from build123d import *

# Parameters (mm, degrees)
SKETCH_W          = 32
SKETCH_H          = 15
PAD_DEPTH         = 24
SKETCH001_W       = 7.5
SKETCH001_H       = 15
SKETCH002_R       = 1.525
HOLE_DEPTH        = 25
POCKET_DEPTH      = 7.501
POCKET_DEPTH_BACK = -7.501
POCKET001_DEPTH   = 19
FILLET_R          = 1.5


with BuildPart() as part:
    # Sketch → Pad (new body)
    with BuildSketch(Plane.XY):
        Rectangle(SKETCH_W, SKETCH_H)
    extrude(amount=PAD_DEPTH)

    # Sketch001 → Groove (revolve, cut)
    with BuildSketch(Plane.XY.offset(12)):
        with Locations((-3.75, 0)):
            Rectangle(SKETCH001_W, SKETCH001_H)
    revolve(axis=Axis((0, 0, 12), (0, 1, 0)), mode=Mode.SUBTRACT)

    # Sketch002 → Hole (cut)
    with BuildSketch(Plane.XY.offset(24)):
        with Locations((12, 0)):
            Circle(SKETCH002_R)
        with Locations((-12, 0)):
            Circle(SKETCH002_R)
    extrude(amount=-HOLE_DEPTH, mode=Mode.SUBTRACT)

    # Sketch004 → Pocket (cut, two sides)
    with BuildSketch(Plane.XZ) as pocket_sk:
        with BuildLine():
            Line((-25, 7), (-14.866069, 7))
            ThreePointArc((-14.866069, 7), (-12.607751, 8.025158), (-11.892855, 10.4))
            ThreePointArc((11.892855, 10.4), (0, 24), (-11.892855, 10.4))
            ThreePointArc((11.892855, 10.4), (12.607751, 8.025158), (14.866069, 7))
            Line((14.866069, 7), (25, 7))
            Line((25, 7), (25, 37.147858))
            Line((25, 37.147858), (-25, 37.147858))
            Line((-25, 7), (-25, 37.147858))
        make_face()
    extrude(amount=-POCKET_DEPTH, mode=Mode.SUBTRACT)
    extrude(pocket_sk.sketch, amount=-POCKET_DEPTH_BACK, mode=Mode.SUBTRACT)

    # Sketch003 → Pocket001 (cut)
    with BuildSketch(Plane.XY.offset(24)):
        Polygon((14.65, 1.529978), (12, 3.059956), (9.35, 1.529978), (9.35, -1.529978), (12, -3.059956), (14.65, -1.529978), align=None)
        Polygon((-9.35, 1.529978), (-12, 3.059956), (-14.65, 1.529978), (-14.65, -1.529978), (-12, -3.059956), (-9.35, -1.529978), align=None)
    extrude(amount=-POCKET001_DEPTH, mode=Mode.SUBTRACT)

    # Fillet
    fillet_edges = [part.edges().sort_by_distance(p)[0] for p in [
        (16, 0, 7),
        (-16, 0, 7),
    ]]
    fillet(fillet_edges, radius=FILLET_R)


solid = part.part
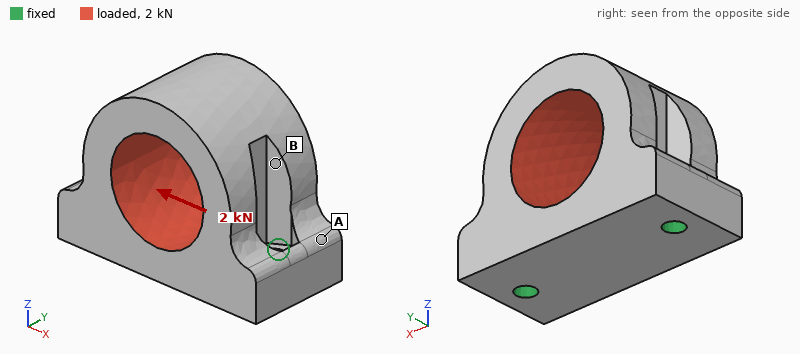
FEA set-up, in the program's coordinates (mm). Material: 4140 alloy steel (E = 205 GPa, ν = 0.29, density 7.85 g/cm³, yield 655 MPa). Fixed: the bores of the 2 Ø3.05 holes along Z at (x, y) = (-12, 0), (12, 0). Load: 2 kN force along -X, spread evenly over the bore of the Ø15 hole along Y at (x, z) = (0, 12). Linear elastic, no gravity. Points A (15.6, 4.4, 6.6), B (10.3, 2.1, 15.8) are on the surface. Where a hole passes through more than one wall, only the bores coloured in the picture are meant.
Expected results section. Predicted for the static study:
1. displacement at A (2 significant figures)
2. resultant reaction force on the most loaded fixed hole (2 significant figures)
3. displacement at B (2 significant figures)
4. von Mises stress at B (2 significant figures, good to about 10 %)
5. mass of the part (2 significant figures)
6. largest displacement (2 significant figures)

1.4 µm
1.2 kN
5.9 µm
17 MPa
43 g
7.1 µm
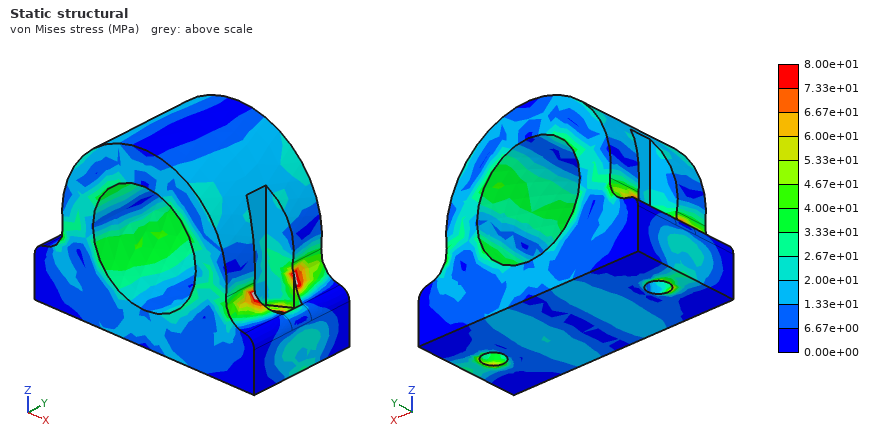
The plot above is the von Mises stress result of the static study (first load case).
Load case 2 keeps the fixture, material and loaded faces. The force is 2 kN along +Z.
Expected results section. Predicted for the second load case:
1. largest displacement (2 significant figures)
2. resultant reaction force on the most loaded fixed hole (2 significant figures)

2.1 µm
1.0 kN
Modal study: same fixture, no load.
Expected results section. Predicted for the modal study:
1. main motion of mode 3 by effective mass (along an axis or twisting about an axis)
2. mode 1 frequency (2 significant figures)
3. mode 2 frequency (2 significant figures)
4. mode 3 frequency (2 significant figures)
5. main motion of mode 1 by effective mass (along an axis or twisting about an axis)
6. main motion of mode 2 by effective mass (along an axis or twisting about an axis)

twisting about Z
10 kHz
17 kHz
22 kHz
along Y
along X
